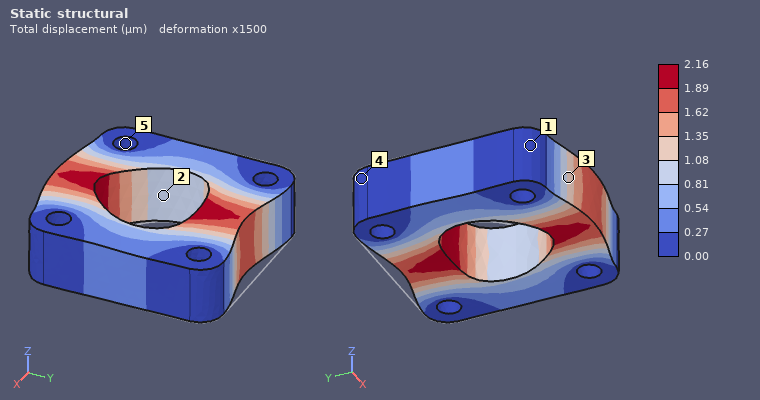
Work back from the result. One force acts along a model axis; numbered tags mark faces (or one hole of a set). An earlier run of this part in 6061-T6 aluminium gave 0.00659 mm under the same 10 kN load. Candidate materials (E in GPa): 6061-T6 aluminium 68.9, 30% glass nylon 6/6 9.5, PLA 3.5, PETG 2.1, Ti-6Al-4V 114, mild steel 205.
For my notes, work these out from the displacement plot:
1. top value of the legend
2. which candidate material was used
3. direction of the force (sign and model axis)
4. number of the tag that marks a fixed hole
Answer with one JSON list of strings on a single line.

["2.16 µm", "mild steel", "-Y", "5"]
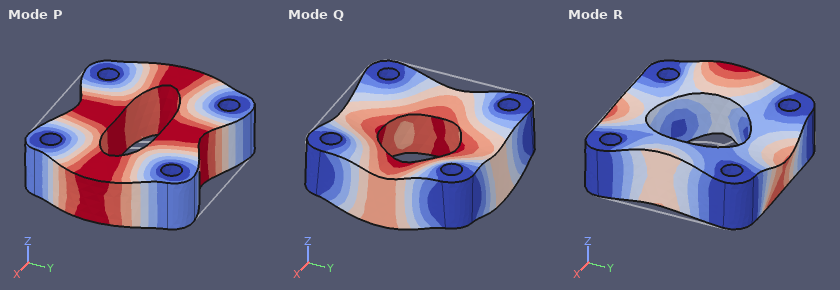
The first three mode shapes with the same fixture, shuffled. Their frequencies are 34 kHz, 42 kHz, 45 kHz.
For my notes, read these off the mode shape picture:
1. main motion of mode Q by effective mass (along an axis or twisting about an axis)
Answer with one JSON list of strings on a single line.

["along Z"]
